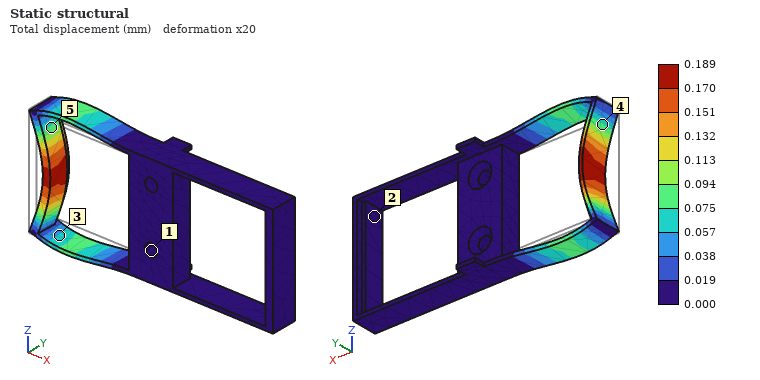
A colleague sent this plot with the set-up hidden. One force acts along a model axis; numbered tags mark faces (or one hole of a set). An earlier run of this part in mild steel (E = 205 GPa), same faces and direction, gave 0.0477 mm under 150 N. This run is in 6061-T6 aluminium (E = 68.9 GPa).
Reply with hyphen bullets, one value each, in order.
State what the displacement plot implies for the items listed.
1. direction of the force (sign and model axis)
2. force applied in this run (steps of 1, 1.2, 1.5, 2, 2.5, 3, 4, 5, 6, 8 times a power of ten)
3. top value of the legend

- +X
- 200 N
- 0.189 mm
